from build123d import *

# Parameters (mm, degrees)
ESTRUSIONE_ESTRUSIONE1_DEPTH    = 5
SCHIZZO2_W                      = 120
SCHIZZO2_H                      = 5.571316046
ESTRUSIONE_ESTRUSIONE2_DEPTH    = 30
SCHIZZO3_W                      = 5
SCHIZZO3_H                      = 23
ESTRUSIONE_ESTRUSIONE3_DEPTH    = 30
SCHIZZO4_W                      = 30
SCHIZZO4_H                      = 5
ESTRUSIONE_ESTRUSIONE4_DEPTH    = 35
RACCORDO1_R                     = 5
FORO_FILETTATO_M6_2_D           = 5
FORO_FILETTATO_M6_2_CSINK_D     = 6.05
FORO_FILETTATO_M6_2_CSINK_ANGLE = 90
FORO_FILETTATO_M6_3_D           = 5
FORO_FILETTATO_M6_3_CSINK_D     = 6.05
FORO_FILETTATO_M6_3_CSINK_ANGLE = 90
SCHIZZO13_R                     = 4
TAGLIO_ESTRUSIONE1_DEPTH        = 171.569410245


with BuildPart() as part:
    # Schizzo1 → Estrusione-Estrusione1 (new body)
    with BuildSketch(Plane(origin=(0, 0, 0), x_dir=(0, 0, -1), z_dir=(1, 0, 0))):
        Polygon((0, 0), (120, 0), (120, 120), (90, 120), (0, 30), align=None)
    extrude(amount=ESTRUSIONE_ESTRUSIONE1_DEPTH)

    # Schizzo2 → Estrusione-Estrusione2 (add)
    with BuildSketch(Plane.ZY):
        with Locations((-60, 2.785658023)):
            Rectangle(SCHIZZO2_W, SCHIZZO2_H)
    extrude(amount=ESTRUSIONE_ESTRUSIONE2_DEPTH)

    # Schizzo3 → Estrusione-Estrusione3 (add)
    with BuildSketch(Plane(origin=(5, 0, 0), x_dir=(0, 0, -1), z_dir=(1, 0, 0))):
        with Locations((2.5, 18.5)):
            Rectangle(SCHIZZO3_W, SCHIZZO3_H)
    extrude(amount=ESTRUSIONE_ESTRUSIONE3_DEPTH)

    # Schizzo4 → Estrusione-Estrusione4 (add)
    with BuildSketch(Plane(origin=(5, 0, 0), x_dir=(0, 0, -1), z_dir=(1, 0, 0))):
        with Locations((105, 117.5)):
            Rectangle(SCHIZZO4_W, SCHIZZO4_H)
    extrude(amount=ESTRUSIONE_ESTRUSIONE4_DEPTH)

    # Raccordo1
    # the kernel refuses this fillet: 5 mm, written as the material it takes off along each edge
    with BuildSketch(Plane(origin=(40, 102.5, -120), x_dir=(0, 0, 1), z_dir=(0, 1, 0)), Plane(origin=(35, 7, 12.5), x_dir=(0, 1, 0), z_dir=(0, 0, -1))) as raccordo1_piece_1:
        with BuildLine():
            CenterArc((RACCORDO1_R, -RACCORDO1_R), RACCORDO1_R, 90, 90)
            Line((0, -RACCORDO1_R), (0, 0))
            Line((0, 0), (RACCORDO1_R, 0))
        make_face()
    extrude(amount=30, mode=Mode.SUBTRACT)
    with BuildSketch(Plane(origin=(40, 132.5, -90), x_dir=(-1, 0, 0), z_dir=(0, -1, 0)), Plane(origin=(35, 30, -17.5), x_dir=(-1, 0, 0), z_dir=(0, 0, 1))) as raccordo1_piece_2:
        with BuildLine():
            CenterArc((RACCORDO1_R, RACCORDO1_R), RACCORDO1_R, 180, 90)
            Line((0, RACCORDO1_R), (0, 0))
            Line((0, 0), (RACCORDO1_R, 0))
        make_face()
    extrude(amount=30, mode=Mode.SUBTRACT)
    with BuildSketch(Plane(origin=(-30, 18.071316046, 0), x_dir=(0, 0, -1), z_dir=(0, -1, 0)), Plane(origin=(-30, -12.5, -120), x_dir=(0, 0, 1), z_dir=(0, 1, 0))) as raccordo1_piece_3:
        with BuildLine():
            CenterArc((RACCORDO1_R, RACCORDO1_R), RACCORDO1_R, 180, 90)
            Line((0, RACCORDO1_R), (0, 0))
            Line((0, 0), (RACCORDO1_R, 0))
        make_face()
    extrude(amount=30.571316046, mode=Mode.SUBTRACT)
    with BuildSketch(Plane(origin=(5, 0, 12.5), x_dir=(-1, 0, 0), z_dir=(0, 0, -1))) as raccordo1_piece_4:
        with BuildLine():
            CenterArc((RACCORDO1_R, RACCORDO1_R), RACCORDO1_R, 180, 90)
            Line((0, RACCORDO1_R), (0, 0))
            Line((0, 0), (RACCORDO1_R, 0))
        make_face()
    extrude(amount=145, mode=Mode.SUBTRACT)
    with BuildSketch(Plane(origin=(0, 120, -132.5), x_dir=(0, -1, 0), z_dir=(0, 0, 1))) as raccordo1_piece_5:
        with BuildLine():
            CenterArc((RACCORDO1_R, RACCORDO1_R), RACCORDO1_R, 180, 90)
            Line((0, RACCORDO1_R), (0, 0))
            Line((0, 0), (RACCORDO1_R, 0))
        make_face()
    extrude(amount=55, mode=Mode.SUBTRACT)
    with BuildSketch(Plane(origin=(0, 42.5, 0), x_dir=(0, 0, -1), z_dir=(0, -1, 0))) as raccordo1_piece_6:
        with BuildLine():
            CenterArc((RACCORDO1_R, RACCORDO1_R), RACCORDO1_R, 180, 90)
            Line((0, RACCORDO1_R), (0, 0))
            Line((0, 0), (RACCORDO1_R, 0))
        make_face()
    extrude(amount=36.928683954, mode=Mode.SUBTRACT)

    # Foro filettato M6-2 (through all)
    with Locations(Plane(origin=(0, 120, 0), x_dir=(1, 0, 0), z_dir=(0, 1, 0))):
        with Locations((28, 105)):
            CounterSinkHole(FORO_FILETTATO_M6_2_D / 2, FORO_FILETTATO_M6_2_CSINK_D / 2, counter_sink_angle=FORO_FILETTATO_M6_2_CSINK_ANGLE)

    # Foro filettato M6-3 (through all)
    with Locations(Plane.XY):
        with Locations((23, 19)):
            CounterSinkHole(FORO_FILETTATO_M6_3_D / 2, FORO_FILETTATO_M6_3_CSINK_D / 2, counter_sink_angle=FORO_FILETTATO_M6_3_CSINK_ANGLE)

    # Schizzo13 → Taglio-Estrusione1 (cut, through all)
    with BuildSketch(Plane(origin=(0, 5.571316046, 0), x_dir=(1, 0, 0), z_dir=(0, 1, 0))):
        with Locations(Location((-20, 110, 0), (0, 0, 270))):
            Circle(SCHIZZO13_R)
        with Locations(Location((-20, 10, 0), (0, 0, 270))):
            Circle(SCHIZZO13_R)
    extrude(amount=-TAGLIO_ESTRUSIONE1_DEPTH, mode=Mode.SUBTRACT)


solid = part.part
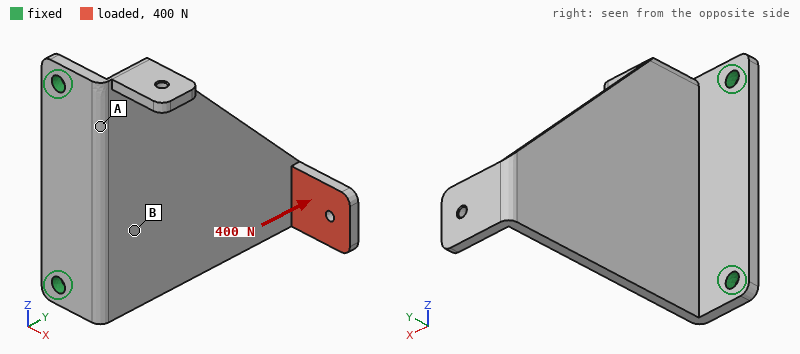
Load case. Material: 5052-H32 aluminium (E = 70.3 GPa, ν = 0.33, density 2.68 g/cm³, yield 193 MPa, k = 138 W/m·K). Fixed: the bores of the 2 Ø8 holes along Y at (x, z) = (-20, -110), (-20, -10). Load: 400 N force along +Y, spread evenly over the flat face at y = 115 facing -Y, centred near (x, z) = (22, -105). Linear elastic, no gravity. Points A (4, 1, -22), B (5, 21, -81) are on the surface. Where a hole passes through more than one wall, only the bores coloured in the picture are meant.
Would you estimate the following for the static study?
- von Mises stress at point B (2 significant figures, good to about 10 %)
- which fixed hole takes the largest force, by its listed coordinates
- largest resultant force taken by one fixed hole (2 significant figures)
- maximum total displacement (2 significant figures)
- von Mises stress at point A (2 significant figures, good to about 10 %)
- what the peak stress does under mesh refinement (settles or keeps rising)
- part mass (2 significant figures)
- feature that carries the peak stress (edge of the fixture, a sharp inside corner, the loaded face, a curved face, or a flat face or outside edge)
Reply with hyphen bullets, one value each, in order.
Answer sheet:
- 16 MPa
- (-20, -110)
- 380 N
- 1.6 mm
- 7.2 MPa
- keeps rising
- 210 g
- edge of the fixture
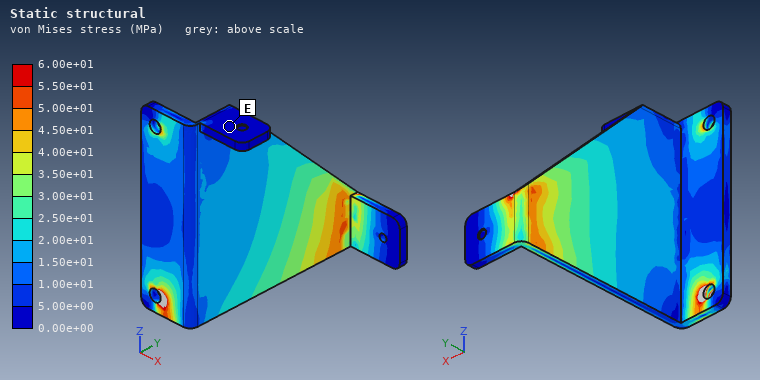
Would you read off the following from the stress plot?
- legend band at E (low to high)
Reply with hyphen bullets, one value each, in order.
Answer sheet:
- 0.00e+00 to 5.00e+00 MPa
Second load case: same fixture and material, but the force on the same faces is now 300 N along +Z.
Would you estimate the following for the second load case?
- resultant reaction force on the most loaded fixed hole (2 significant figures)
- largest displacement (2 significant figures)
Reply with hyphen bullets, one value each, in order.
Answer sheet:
- 410 N
- 0.45 mm
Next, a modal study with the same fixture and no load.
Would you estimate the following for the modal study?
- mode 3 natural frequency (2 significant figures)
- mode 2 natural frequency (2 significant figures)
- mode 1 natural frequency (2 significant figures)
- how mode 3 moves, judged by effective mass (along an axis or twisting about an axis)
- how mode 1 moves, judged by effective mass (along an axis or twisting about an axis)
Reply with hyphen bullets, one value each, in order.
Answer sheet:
- 1300 Hz
- 950 Hz
- 250 Hz
- along Z
- along X
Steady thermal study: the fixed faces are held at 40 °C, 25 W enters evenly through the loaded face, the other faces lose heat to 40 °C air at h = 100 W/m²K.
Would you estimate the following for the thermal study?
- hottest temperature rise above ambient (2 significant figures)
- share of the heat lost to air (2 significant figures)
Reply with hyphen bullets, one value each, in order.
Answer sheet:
- 46 K
- 88 %
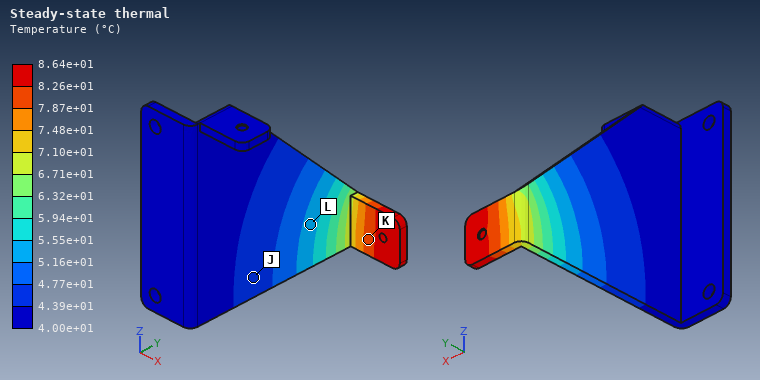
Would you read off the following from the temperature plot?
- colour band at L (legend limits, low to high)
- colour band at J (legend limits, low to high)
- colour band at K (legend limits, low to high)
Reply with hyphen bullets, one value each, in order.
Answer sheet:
- 5.16e+01 to 5.55e+01 °C
- 4.39e+01 to 4.77e+01 °C
- 7.87e+01 to 8.26e+01 °C
